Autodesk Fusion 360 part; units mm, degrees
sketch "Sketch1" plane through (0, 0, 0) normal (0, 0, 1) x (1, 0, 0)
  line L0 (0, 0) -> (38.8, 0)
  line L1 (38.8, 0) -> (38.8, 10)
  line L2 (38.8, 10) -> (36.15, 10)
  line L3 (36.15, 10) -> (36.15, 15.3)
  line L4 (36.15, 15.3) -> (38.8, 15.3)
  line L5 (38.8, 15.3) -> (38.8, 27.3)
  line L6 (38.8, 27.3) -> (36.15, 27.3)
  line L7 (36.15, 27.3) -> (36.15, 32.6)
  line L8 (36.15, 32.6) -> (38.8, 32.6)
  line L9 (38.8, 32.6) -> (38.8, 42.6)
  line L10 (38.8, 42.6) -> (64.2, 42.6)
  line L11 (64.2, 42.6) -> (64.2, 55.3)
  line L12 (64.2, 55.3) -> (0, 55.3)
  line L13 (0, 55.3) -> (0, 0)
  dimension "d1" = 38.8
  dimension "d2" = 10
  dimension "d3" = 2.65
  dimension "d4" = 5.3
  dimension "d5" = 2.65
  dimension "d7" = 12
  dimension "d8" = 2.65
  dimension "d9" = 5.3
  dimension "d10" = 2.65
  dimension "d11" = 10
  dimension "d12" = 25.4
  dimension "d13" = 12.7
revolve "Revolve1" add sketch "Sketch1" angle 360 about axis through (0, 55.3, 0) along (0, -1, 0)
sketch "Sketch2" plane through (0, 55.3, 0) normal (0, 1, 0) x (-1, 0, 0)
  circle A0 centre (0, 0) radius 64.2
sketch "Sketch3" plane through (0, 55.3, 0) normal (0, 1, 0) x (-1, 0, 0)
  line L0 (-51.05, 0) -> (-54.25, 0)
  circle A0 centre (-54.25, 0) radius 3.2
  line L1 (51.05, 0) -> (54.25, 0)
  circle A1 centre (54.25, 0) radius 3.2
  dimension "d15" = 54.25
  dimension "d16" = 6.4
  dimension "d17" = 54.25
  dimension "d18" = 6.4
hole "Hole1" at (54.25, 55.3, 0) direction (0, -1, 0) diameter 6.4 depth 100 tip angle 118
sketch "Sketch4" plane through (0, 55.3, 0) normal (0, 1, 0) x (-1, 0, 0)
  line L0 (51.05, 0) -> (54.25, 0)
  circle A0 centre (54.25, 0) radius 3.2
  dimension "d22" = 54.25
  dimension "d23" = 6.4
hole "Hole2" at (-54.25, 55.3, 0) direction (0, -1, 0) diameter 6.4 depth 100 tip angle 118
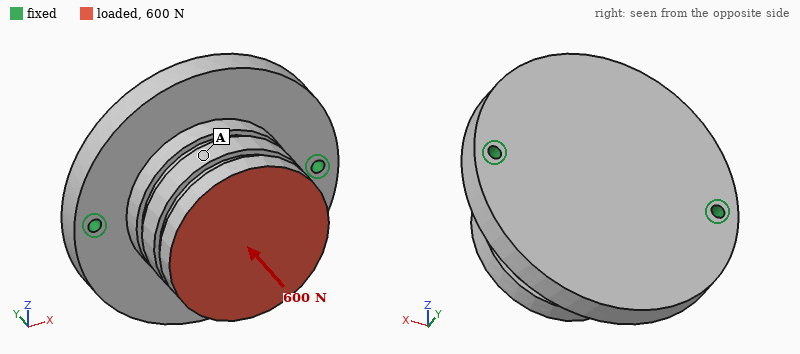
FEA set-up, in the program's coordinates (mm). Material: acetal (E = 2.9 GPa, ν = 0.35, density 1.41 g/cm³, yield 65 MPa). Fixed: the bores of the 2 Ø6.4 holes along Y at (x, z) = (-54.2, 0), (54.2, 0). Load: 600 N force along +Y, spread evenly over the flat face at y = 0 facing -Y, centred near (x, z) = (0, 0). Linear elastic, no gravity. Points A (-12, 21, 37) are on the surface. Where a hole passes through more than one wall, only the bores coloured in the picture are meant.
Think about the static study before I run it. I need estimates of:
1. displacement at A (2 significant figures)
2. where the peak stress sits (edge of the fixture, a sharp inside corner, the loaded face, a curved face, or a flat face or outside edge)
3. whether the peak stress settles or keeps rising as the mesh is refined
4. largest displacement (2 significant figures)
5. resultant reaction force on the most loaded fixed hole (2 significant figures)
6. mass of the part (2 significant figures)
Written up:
39 µm
edge of the fixture
keeps rising
46 µm
320 N
510 g
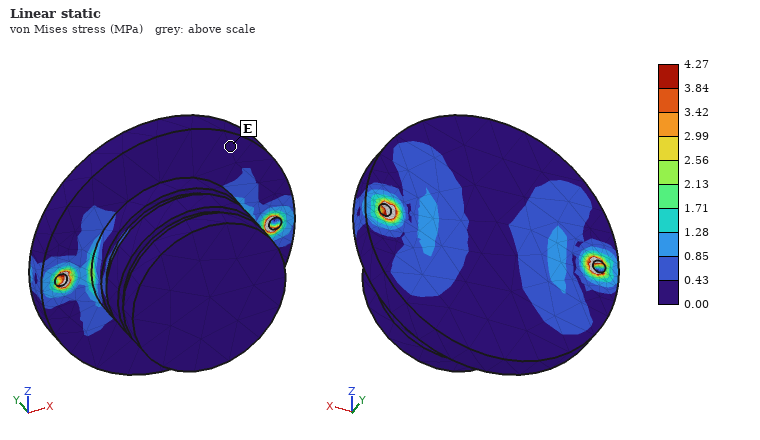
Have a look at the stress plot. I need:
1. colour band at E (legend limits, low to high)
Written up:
0.00 to 0.43 MPa
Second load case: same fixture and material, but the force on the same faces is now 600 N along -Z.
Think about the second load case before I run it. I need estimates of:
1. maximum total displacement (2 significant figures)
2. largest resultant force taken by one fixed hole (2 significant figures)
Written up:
0.68 mm
300 N
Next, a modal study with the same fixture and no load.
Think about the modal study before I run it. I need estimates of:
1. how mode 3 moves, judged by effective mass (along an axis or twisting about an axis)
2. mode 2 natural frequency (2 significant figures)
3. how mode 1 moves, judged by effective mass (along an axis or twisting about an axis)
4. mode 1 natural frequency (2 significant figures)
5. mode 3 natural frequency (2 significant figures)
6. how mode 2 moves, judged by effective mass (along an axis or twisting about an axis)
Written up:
along X
910 Hz
along Z
350 Hz
1300 Hz
along Y
